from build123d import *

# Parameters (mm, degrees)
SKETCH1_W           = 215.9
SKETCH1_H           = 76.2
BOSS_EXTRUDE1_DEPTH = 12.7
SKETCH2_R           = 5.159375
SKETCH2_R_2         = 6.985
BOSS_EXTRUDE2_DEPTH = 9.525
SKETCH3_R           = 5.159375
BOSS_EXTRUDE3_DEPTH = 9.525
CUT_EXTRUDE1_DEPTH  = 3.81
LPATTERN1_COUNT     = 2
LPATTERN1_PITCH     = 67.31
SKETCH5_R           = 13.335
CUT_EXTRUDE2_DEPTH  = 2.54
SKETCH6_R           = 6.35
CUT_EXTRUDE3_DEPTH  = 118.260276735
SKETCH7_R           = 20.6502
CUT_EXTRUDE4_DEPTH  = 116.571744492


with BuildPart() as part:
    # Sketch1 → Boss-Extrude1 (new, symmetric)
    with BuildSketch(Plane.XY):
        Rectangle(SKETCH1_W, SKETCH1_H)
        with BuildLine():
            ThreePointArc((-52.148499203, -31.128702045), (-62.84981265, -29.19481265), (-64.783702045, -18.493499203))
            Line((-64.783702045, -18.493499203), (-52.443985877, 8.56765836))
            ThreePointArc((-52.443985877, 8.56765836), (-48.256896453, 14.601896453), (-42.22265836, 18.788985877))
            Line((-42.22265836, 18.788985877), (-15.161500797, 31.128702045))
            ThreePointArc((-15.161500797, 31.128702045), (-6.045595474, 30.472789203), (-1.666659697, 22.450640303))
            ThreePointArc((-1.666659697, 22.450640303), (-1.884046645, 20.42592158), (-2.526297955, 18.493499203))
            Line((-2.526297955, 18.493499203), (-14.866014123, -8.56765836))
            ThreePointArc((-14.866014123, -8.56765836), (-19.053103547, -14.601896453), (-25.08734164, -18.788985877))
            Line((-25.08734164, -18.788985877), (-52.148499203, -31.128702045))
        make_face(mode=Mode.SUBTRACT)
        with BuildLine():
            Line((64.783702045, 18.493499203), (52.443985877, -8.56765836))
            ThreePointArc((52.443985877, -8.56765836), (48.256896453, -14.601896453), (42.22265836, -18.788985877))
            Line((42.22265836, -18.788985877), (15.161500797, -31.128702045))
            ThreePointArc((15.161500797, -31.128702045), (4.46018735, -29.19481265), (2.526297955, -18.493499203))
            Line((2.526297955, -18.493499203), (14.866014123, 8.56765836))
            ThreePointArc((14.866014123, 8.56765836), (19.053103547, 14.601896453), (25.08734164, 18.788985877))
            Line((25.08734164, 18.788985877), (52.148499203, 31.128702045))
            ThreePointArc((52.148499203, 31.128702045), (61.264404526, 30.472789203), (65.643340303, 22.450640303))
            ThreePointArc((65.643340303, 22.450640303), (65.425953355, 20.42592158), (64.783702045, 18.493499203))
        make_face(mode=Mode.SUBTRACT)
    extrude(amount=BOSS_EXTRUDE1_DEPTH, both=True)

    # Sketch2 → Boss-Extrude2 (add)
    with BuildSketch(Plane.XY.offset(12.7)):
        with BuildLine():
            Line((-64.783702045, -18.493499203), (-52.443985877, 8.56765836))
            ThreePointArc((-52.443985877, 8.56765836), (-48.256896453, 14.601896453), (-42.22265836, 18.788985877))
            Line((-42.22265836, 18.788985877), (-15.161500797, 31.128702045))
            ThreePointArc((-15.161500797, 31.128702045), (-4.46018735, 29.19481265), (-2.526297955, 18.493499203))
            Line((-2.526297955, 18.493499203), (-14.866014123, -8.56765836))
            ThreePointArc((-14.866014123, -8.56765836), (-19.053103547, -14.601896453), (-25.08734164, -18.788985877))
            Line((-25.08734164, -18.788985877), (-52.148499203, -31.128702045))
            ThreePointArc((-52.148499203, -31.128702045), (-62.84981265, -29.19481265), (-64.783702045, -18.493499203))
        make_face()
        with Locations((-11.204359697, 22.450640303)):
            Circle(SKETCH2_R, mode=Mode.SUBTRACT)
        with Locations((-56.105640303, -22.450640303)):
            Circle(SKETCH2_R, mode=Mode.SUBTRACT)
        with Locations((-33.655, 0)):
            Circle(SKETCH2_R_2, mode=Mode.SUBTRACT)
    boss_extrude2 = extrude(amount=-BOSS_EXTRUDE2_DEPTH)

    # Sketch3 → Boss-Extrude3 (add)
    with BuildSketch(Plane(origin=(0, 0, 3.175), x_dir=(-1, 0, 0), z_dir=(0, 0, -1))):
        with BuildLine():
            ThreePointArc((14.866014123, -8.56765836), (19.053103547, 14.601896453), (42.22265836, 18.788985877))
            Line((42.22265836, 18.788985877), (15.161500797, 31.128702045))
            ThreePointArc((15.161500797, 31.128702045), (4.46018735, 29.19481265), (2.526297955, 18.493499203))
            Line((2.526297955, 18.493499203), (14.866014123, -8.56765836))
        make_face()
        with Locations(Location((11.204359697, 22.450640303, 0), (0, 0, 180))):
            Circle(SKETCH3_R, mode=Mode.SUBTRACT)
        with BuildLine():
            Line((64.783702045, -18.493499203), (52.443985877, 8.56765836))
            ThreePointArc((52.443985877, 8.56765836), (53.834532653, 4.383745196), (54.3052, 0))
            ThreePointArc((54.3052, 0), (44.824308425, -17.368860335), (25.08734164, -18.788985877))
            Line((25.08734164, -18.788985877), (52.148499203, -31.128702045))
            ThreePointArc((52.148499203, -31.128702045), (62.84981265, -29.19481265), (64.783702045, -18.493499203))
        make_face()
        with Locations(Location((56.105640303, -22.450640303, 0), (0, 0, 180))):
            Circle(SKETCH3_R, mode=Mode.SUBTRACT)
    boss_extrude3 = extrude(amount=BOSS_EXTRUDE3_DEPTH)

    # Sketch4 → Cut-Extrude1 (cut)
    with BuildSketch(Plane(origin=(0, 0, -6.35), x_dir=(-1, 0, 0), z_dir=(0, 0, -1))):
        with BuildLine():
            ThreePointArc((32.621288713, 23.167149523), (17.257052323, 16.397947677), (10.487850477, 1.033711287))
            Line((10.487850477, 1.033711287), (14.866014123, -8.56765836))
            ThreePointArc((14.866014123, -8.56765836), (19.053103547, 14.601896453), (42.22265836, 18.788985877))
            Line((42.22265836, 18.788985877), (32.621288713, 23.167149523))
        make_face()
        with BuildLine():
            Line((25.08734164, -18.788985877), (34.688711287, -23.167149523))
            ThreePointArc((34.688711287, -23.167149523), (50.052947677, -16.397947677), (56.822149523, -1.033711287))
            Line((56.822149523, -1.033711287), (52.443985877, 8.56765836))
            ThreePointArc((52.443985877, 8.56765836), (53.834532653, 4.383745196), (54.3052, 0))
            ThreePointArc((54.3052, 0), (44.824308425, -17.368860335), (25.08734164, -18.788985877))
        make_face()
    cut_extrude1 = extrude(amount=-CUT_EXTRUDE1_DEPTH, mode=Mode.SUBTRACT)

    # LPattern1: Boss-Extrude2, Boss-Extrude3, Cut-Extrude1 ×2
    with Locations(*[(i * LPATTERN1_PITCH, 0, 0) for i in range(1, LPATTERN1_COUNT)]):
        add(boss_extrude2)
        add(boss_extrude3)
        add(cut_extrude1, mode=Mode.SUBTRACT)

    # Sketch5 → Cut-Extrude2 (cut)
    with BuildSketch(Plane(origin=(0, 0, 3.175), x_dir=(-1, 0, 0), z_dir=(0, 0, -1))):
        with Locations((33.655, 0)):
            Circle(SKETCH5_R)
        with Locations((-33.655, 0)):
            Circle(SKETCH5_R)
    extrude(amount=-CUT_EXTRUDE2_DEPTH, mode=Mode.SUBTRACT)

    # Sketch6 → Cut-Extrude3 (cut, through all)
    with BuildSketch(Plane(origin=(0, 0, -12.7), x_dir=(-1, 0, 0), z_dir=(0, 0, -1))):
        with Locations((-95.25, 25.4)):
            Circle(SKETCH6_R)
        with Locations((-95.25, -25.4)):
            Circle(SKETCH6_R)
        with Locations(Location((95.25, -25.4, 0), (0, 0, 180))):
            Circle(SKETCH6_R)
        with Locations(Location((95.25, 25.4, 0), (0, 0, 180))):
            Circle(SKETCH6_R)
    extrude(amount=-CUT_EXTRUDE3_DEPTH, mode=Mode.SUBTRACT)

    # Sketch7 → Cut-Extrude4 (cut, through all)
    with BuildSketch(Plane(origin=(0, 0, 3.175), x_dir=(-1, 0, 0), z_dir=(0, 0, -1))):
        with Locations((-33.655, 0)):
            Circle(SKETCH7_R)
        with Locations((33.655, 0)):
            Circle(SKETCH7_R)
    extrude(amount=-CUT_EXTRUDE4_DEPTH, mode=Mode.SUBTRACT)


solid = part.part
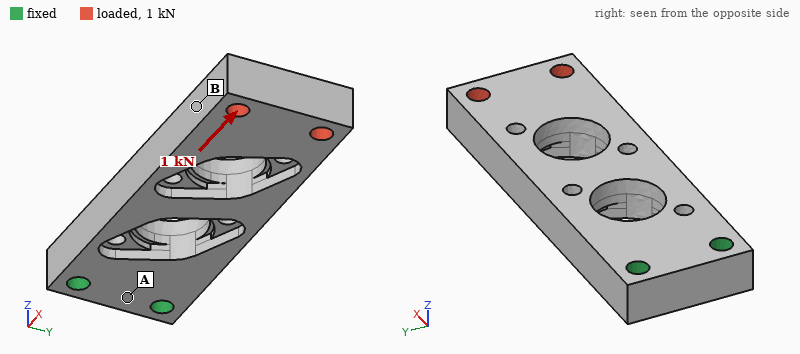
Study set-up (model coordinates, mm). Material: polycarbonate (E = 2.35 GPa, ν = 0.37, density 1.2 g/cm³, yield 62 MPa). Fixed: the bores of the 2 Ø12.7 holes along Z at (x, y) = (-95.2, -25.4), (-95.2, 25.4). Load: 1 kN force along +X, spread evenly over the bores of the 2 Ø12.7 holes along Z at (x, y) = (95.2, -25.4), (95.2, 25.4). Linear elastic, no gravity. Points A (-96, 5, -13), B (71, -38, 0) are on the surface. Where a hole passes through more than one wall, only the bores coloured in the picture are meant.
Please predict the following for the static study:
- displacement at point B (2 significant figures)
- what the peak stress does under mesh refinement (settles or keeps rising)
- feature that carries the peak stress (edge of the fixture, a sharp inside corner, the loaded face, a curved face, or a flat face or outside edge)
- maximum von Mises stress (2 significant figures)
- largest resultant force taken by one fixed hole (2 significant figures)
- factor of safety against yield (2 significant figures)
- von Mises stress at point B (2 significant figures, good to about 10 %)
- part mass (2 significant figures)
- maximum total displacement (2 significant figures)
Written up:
0.16 mm
settles
a curved face
4.2 MPa
500 N
15
1.1 MPa
380 g
0.23 mm
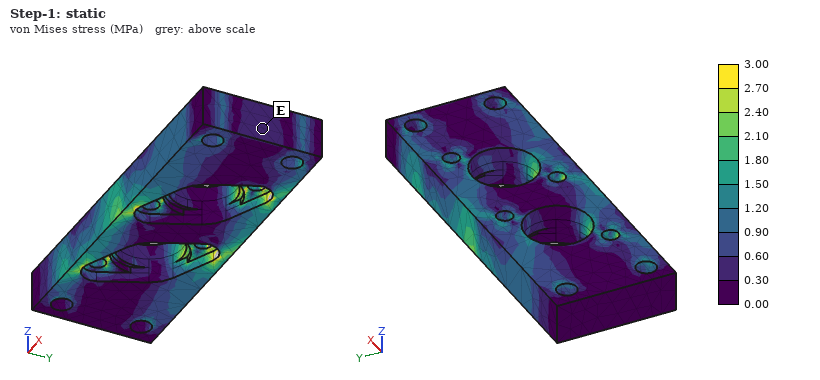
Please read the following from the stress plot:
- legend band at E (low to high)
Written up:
0.30 to 0.60 MPa
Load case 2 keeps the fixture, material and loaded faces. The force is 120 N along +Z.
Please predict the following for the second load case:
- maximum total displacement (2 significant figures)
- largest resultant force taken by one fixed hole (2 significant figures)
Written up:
2.5 mm
67 N
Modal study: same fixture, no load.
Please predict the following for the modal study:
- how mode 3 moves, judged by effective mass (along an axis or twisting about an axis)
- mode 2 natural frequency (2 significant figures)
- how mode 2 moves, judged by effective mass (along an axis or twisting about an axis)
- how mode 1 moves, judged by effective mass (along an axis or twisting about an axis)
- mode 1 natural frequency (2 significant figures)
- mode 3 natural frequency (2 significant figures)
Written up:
twisting about X
340 Hz
along Y
along Z
110 Hz
470 Hz
